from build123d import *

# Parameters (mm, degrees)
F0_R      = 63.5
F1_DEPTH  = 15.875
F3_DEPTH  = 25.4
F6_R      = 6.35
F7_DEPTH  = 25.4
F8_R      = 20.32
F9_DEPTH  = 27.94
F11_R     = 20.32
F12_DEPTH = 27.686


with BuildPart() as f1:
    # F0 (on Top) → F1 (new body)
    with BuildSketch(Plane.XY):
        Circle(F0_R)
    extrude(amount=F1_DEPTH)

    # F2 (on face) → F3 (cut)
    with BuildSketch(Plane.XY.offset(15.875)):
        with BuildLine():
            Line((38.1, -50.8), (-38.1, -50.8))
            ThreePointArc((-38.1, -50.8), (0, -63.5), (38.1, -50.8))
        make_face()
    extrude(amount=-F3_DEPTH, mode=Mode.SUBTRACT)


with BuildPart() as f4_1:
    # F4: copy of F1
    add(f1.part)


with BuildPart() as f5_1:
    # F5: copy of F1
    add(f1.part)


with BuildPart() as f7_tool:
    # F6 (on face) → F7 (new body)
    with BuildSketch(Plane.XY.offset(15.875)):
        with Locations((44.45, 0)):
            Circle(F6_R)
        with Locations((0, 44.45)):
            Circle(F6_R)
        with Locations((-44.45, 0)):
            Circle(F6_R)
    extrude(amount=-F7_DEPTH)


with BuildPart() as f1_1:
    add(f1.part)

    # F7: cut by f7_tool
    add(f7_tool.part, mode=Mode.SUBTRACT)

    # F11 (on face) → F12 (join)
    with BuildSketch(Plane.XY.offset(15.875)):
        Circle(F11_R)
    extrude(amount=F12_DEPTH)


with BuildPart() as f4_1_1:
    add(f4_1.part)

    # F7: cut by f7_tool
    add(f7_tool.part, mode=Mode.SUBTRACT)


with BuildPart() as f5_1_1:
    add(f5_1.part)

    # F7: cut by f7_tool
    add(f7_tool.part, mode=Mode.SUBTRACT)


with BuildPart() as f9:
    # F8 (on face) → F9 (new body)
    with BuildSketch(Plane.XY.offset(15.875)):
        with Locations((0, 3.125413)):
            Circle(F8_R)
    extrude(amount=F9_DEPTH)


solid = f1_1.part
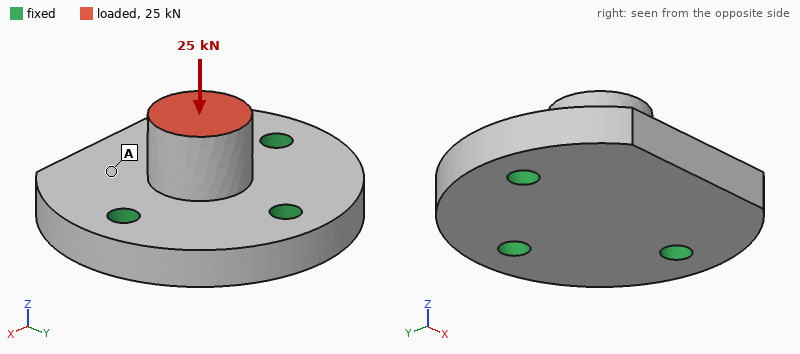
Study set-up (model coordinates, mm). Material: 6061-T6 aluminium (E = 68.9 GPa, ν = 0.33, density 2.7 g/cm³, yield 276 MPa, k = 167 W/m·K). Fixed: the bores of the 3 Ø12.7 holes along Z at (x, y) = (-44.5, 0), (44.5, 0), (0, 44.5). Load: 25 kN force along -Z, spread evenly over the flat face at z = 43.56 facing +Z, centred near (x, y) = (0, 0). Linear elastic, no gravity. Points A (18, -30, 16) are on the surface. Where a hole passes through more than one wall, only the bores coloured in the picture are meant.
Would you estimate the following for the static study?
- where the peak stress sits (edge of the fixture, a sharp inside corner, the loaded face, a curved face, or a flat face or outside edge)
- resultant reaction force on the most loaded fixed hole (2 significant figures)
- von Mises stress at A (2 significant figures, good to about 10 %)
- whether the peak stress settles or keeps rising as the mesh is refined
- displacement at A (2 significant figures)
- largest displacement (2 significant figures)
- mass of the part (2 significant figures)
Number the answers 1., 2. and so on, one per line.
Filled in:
1. edge of the fixture
2. 10 kN
3. 17 MPa
4. keeps rising
5. 51 µm
6. 74 µm
7. 600 g
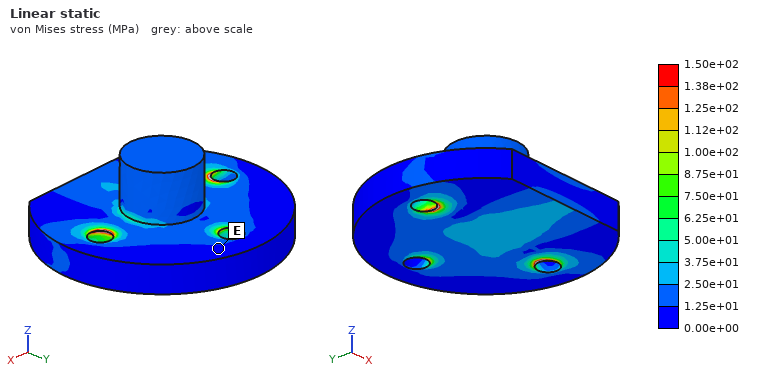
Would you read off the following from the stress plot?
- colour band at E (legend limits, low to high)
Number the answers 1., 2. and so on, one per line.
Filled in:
1. 0.00e+00 to 1.25e+01 MPa
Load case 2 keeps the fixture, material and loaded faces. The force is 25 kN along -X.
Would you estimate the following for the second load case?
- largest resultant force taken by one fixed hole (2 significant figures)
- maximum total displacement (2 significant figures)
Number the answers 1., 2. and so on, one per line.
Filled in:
1. 16 kN
2. 0.12 mm
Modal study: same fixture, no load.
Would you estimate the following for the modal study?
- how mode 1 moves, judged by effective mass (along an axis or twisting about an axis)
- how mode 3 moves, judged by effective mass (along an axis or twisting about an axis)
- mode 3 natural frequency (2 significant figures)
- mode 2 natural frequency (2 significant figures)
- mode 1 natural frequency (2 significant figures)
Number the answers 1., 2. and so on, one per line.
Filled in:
1. along Z
2. along Z
3. 10 kHz
4. 8500 Hz
5. 4500 Hz
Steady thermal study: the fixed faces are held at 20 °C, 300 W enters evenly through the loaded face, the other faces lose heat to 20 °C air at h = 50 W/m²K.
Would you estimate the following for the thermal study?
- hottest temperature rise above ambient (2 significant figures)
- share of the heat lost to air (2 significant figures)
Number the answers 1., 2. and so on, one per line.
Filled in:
1. 66 K
2. 6.9 %
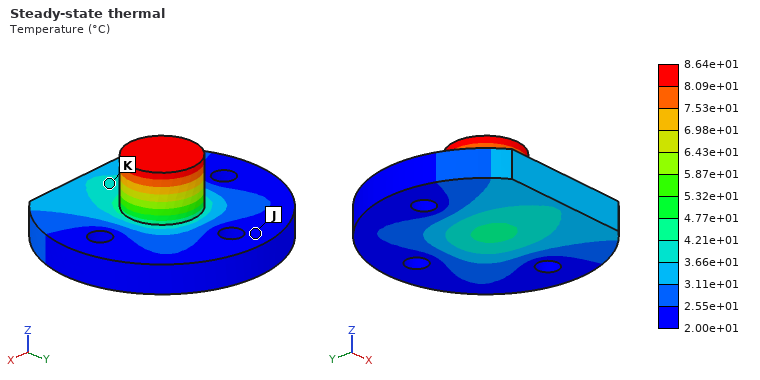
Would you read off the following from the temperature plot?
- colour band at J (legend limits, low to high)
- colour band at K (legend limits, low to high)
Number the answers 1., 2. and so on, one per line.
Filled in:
1. 2.00e+01 to 2.55e+01 °C
2. 3.66e+01 to 4.21e+01 °C
